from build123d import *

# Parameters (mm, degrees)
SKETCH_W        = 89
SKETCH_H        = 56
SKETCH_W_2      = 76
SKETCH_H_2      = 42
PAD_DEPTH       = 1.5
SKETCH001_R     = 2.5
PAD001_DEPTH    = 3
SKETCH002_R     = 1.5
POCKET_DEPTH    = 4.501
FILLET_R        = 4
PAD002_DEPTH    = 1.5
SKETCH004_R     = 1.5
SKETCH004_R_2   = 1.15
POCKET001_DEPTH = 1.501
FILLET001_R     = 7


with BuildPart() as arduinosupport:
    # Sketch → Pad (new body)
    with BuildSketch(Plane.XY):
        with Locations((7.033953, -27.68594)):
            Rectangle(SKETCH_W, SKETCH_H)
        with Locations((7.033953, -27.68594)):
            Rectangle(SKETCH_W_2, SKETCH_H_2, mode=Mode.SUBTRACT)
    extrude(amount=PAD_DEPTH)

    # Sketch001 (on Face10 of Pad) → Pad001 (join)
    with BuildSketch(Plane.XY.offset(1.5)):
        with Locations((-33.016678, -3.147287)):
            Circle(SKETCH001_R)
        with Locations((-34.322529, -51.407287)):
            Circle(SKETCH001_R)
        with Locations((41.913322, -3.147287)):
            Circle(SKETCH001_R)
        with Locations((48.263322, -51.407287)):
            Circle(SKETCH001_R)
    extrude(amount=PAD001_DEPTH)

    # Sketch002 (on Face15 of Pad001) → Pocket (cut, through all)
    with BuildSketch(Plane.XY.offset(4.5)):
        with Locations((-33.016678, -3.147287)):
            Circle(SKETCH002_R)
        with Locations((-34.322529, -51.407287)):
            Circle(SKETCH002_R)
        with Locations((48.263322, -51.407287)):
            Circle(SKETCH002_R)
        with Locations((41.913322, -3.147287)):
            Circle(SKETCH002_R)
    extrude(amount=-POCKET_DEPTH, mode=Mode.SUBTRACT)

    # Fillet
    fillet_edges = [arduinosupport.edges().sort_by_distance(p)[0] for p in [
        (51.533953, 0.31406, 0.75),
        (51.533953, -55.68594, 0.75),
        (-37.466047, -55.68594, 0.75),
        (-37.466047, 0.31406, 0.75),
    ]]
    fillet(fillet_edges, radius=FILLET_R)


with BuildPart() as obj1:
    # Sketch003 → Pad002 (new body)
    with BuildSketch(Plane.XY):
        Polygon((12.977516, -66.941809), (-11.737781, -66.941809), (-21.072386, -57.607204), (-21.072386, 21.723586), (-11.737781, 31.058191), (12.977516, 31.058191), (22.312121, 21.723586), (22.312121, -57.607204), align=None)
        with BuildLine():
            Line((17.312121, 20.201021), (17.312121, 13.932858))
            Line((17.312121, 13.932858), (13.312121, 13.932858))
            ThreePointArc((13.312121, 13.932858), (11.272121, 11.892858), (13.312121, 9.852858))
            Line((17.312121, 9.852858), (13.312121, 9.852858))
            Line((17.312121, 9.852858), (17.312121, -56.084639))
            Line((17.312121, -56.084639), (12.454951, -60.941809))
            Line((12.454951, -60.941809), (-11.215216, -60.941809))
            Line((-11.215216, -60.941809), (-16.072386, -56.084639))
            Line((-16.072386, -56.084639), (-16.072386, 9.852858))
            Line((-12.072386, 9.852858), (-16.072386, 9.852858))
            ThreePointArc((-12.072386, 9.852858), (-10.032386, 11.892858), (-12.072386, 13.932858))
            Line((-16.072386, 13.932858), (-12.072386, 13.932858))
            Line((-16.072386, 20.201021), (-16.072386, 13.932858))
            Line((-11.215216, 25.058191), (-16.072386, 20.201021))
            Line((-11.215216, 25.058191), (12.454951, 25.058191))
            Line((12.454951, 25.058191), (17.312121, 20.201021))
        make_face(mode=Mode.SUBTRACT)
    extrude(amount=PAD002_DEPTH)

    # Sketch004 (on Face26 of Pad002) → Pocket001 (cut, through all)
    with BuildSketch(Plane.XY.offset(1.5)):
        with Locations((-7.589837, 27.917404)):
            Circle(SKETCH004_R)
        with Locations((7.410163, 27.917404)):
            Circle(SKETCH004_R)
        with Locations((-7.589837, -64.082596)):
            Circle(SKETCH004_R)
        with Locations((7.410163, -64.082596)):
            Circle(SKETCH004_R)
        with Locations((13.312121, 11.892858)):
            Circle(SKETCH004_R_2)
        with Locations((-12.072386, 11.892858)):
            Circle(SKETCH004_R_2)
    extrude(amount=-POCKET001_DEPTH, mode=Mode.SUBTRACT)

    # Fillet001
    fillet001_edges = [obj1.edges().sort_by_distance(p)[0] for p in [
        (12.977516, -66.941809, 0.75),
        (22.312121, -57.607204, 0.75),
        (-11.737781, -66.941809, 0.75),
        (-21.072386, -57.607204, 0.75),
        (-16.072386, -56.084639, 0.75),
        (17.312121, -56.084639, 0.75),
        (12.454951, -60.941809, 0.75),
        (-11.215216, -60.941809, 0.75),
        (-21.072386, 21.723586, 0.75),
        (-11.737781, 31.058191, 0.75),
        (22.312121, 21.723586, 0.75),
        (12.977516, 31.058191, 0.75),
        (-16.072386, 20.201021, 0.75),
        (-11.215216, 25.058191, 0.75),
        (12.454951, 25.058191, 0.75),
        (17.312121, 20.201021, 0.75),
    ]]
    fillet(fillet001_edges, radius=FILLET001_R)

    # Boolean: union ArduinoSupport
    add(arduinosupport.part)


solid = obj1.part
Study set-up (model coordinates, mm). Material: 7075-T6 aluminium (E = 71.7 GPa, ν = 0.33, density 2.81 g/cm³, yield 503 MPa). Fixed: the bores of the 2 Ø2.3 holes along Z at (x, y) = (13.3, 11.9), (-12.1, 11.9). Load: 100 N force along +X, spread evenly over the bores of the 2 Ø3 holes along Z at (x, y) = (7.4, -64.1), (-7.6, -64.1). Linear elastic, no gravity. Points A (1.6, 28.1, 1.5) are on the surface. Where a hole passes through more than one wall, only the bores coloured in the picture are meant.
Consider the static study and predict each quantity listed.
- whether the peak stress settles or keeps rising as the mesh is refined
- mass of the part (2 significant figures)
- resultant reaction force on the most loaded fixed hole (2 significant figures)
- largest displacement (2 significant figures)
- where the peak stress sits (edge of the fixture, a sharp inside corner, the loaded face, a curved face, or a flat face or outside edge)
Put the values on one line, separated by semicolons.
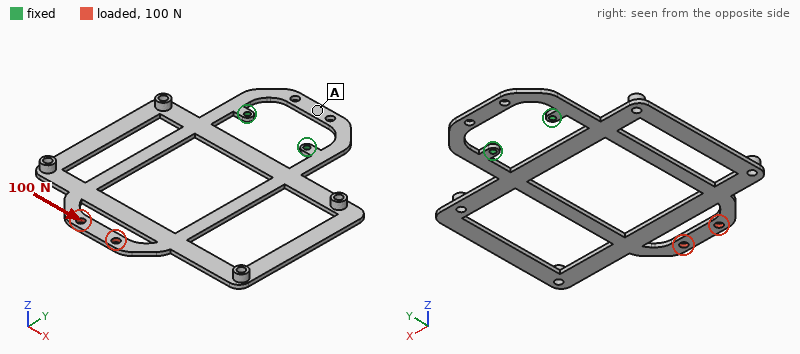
keeps rising; 13 g; 210 N; 0.64 mm; edge of the fixture
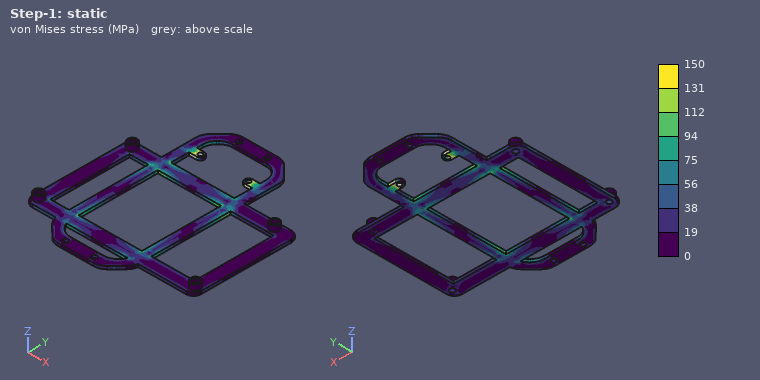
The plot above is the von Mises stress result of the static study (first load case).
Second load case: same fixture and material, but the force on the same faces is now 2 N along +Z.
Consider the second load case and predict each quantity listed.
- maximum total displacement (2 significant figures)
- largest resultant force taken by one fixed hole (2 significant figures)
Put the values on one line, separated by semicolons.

1.3 mm; 1.0 N
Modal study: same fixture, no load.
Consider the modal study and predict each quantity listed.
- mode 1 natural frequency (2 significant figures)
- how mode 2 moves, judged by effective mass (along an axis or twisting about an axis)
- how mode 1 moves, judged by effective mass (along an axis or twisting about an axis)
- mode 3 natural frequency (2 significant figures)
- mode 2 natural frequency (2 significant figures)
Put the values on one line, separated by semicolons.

110 Hz; twisting about Y; along Z; 610 Hz; 260 Hz
